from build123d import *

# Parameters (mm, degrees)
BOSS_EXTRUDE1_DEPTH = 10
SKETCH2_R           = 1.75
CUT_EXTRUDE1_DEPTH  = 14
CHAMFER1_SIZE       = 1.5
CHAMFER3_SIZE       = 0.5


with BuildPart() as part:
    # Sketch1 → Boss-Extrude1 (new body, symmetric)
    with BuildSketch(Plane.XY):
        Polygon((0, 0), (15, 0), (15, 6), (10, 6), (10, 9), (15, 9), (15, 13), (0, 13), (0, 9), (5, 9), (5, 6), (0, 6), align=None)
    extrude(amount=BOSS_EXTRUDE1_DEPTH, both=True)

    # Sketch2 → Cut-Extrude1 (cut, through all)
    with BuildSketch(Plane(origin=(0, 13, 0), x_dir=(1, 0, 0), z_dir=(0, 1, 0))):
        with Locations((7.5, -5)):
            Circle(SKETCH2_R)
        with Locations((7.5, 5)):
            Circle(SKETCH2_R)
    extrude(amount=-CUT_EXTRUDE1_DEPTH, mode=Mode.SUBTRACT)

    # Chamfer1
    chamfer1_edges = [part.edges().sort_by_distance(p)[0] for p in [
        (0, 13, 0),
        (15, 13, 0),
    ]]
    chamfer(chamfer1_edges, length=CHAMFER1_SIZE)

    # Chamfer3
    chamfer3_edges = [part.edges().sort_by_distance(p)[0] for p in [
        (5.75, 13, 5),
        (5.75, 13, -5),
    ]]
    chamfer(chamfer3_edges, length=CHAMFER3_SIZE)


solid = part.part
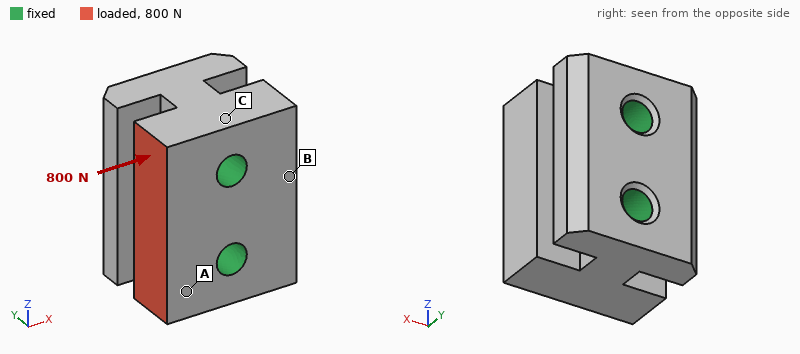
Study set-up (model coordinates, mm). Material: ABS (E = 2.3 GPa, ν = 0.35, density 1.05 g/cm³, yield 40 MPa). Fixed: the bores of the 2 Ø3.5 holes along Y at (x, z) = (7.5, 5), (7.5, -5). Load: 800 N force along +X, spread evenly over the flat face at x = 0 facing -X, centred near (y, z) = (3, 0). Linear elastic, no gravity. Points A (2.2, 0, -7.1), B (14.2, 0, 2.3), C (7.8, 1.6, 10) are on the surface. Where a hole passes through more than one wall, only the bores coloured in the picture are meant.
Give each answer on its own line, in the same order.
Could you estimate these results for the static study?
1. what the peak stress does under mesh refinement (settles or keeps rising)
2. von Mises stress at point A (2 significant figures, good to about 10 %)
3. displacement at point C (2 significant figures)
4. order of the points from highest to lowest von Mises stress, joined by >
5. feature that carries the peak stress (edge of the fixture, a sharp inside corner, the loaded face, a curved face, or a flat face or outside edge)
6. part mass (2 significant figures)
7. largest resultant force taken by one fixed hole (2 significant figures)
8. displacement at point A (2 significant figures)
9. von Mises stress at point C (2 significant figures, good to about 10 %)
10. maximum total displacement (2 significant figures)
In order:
keeps rising
7.0 MPa
10 µm
A > C > B
edge of the fixture
3.2 g
400 N
20 µm
4.1 MPa
32 µm
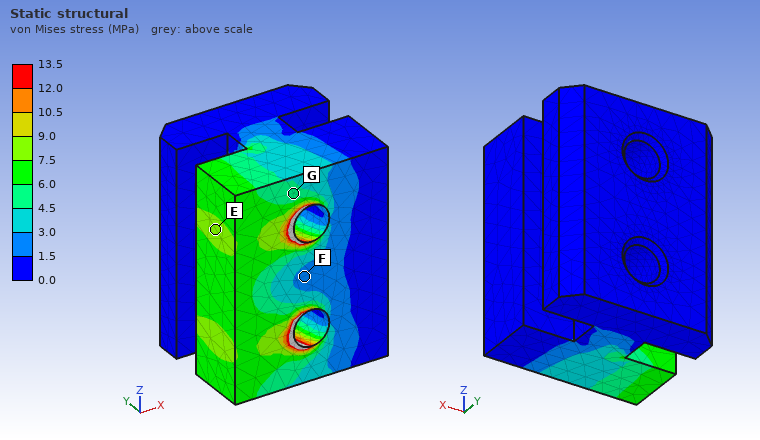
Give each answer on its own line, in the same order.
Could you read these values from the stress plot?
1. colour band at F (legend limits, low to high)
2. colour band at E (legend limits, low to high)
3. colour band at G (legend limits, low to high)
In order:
1.5 to 3.0 MPa
7.5 to 9.0 MPa
4.5 to 6.0 MPa
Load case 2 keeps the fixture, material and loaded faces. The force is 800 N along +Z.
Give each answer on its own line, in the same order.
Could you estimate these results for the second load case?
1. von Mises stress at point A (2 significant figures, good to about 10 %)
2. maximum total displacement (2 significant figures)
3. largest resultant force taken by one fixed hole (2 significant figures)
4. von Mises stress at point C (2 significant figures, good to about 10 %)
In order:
8.8 MPa
0.12 mm
570 N
10 MPa
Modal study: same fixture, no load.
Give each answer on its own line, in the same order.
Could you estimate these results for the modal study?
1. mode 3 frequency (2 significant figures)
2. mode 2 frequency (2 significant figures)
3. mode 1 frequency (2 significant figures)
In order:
21 kHz
21 kHz
19 kHz
